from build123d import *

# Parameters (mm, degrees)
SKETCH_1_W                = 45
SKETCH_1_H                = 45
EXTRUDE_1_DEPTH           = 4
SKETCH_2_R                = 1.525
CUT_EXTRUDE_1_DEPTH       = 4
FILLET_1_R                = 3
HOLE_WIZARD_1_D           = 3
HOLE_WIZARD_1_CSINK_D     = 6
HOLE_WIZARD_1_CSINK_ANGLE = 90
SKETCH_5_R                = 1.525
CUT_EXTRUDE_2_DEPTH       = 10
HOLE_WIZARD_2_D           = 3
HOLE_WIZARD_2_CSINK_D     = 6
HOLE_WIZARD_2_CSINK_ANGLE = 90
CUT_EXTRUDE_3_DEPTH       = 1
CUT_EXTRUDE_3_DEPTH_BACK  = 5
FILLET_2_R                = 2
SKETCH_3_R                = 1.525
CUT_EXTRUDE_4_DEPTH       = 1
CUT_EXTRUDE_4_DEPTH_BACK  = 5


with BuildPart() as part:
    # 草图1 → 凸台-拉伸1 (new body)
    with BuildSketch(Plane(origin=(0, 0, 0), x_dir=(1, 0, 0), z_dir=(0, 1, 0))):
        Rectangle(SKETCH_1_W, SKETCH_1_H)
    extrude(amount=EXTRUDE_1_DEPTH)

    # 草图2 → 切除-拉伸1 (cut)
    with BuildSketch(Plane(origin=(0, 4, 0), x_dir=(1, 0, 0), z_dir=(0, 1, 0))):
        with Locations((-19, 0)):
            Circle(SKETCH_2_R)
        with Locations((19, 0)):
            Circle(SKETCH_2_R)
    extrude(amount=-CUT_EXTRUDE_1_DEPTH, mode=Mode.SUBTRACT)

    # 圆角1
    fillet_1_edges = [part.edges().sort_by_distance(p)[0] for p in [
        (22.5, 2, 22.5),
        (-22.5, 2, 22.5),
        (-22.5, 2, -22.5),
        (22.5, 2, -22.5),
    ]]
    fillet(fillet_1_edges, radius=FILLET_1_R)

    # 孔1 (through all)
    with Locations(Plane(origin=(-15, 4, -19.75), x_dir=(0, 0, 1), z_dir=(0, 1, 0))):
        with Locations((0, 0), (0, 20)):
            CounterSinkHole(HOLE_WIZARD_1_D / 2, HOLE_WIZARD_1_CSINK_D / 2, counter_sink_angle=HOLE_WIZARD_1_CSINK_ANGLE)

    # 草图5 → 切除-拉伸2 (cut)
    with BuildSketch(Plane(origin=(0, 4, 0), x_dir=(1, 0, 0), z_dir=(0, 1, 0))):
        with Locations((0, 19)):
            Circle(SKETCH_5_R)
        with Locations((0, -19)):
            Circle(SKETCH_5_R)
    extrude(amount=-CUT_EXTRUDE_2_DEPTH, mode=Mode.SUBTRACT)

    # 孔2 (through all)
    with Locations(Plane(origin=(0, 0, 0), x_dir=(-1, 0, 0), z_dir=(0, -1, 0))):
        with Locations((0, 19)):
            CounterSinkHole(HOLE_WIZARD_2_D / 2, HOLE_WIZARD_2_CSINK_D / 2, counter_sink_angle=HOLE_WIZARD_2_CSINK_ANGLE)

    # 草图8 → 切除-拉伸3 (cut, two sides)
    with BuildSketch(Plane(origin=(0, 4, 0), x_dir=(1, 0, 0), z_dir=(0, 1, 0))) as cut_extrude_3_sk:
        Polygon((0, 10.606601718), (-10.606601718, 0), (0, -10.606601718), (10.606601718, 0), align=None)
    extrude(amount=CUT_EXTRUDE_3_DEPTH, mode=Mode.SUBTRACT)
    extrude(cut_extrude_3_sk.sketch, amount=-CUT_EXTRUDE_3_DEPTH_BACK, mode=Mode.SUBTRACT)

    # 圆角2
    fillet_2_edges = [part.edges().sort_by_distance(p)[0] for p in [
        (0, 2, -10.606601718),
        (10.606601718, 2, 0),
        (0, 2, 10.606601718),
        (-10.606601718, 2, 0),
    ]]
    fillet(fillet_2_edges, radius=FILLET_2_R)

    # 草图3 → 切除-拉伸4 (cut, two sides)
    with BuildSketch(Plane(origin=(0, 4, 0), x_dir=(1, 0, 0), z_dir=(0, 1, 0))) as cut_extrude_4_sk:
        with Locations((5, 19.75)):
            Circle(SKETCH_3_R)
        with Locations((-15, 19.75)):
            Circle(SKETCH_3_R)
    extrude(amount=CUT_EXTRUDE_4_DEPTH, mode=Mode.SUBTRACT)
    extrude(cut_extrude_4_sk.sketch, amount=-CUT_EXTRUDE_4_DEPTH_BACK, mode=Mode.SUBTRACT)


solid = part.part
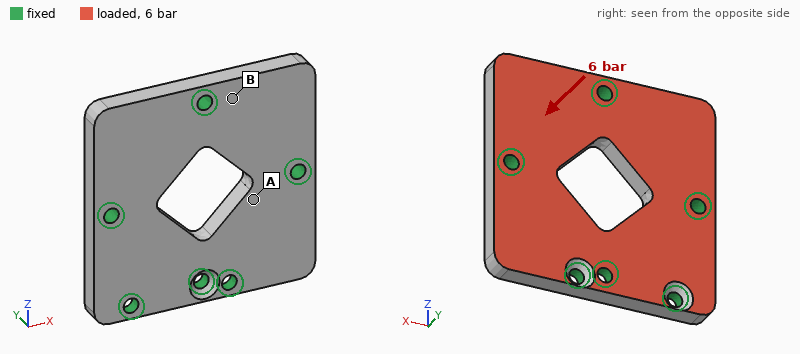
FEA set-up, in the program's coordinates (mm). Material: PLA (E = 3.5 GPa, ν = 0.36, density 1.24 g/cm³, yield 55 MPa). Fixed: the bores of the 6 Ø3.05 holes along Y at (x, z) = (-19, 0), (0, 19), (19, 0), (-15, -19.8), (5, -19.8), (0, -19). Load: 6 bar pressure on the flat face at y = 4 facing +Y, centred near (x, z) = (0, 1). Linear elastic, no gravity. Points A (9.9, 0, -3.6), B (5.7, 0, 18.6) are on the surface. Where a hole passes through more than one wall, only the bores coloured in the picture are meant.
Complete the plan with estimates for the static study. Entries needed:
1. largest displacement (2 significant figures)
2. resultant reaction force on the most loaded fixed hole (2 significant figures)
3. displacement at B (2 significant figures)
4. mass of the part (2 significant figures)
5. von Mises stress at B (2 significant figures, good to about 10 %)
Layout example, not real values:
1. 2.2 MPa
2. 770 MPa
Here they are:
1. 0.30 mm
2. 270 N
3. 0.052 mm
4. 8.6 g
5. 11 MPa
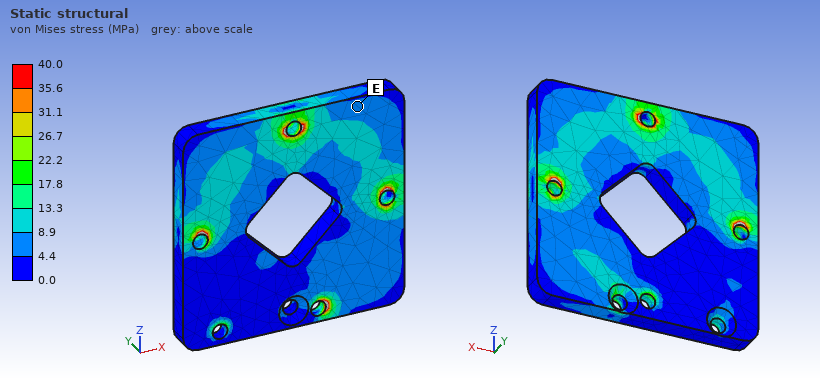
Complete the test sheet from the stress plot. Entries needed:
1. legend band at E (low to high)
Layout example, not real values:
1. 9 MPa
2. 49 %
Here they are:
1. 4.4 to 8.9 MPa
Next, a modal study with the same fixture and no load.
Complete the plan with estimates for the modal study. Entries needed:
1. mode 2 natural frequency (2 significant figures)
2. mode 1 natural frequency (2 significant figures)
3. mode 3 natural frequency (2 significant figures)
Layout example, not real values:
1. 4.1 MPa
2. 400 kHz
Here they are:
1. 4100 Hz
2. 4100 Hz
3. 5000 Hz
